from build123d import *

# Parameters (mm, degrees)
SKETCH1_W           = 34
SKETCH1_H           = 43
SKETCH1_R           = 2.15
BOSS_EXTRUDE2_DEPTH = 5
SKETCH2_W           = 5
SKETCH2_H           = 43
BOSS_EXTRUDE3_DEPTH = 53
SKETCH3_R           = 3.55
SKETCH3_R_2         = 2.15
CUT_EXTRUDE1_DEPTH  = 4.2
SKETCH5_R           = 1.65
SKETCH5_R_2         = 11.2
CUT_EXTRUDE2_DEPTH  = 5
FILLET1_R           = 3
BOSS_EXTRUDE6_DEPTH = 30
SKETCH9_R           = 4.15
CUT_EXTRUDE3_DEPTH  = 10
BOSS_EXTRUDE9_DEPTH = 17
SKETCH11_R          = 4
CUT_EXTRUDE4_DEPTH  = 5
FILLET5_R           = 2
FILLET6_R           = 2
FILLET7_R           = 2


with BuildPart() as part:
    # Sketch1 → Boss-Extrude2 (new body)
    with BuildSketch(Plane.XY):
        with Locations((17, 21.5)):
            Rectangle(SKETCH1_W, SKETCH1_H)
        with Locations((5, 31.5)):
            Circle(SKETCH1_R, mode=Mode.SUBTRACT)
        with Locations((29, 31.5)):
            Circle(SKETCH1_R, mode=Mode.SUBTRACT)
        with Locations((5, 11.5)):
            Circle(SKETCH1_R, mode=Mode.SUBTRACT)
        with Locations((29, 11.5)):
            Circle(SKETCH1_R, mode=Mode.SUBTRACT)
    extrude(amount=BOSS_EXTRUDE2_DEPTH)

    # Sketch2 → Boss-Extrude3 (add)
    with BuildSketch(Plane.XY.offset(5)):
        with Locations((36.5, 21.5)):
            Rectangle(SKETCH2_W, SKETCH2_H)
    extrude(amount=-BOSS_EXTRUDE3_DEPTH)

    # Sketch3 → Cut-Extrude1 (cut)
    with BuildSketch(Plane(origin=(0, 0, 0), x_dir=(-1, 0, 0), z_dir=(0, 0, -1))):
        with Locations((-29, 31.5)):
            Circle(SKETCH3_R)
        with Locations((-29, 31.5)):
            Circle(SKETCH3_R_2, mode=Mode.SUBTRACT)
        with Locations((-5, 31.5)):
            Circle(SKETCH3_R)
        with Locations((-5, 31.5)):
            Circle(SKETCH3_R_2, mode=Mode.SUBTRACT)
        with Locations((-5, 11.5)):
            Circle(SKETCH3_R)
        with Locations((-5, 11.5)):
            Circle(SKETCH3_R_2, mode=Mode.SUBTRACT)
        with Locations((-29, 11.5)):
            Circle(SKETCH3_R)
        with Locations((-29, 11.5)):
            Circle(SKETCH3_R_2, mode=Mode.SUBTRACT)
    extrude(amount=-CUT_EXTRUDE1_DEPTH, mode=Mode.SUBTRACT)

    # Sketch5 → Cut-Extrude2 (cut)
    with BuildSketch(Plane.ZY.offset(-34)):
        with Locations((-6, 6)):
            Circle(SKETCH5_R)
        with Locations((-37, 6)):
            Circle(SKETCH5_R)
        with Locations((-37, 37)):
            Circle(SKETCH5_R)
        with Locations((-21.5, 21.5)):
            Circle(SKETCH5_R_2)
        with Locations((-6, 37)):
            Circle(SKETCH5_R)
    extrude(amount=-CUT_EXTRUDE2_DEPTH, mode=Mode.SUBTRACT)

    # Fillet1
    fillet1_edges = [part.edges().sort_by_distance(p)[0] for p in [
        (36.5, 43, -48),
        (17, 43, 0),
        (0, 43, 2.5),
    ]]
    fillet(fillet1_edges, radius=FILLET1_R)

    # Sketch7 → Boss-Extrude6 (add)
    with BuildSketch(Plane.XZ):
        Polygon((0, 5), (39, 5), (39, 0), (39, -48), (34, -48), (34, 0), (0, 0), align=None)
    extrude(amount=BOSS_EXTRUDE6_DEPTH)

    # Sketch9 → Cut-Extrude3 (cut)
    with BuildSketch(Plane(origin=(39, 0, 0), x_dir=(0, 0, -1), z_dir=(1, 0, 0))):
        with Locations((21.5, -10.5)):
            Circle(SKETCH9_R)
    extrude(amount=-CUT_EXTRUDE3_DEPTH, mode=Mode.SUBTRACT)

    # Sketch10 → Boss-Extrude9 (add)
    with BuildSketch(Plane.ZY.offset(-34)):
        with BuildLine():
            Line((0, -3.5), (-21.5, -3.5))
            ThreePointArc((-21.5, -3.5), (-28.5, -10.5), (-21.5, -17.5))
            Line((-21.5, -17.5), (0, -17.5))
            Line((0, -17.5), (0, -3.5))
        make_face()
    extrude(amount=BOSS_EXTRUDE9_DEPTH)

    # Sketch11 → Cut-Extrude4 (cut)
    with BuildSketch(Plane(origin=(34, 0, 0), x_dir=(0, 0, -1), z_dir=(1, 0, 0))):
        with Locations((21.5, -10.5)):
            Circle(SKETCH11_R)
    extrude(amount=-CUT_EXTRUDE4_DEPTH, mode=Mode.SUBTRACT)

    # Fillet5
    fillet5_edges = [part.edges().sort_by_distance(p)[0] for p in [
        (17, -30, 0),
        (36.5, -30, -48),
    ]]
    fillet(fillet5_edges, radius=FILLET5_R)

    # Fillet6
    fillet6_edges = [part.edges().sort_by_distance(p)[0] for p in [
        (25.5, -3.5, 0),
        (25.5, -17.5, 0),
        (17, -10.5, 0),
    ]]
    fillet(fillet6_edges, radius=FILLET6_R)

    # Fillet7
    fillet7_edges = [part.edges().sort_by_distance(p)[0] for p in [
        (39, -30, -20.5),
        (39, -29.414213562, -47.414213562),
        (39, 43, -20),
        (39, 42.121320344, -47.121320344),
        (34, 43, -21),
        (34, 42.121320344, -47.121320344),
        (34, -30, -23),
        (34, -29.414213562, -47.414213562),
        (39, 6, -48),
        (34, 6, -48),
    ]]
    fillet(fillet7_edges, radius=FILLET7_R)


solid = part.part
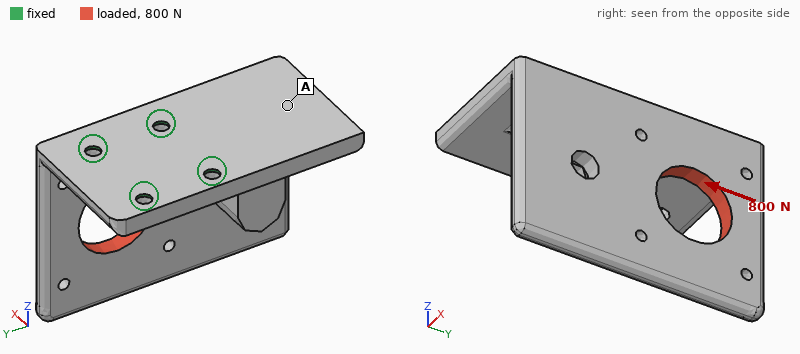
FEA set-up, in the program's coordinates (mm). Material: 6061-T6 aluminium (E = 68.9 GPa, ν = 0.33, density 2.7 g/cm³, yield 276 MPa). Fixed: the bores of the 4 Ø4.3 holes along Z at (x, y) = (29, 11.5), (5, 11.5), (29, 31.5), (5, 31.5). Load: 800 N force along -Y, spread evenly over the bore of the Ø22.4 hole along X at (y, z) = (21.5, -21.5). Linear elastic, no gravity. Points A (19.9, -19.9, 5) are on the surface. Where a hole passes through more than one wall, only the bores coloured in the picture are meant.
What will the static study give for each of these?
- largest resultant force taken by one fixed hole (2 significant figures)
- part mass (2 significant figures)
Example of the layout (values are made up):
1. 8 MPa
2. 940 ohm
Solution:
1. 1.0 kN
2. 93 g
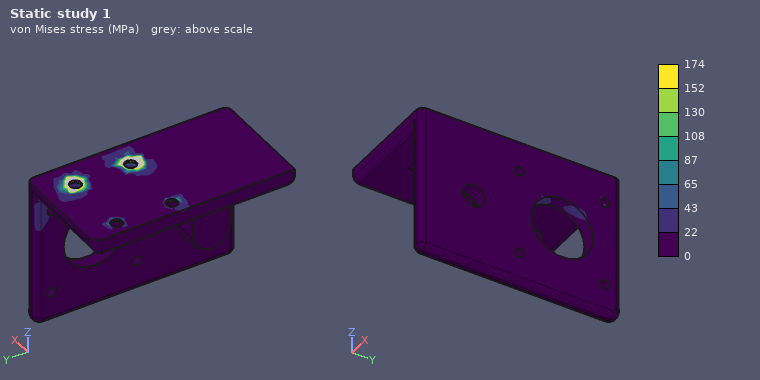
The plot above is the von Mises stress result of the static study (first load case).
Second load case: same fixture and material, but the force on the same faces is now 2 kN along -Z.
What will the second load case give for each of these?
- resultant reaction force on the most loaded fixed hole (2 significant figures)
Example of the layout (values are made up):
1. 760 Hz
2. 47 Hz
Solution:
1. 1.4 kN
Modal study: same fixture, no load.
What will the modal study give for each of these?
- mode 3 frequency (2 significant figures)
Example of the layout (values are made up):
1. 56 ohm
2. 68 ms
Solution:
1. 2900 Hz
